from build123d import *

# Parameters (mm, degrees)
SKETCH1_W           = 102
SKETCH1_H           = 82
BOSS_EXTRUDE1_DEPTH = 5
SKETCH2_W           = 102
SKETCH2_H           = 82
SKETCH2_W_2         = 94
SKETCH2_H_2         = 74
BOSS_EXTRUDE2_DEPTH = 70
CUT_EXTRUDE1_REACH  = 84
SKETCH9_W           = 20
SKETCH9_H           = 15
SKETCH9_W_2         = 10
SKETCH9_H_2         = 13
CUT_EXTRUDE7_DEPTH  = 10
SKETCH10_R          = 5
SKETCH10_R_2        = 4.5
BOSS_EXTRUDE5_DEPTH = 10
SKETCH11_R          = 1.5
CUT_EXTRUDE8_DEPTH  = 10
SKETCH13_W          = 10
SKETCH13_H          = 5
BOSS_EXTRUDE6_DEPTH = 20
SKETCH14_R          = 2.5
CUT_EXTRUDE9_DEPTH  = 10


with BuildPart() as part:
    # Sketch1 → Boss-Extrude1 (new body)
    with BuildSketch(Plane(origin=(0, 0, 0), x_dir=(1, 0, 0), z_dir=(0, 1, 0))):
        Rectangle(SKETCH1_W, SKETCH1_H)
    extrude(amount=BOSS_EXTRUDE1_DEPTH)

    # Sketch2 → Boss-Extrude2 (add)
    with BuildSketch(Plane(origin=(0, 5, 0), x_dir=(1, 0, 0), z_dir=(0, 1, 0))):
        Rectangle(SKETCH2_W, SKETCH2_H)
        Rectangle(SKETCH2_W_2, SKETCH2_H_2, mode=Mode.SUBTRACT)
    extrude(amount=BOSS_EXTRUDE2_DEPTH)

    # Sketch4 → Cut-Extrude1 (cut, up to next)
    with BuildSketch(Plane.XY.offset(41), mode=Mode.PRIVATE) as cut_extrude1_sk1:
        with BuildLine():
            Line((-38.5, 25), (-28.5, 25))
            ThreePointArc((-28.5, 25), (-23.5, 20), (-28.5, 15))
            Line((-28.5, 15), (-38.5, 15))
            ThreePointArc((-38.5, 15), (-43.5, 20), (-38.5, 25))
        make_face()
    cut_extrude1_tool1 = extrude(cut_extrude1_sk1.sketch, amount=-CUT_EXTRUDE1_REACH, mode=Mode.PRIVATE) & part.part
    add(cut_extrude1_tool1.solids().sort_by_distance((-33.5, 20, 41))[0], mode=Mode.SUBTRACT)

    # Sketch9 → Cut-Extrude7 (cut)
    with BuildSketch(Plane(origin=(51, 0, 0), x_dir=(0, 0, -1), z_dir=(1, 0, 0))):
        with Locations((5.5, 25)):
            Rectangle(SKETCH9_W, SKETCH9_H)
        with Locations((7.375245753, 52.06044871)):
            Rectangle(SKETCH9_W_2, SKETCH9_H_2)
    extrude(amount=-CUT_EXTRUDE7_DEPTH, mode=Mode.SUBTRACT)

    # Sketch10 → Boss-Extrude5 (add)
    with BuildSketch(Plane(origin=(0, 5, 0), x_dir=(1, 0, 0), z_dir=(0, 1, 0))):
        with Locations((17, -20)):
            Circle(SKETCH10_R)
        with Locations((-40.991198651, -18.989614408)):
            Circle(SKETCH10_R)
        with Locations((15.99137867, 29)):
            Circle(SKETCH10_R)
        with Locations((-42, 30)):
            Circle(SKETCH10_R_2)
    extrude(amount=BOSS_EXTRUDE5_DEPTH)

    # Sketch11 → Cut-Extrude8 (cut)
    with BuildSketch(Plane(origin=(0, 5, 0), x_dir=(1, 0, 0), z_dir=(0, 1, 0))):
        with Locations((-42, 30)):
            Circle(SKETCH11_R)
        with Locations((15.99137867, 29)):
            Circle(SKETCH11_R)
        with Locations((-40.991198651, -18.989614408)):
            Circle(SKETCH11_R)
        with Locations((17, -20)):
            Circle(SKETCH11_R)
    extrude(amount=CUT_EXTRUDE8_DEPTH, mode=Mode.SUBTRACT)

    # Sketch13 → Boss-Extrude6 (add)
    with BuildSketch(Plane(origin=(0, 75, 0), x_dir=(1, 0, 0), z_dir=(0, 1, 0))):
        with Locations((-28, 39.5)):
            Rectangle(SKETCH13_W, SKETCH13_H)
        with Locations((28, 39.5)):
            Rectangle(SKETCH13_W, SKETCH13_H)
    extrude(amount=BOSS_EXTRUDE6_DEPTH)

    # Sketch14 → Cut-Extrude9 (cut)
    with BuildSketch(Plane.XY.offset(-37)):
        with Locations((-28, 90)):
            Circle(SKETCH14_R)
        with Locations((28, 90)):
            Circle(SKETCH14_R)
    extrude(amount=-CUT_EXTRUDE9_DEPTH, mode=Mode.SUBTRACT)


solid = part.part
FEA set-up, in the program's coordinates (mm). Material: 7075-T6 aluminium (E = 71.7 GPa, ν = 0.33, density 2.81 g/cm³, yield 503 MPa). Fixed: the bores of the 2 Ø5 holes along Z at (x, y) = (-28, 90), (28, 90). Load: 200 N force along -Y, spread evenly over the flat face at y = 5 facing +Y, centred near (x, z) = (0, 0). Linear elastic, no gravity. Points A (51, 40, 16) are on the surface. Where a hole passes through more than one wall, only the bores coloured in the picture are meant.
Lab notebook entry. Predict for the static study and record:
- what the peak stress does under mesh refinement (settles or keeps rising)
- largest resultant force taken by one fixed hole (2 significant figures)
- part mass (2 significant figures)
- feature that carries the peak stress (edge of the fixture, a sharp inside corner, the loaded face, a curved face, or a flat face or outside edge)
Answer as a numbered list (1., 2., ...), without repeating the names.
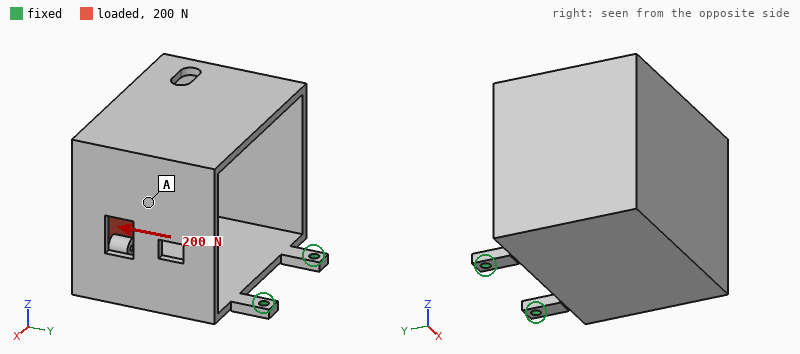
1. keeps rising
2. 100 N
3. 400 g
4. a sharp inside corner
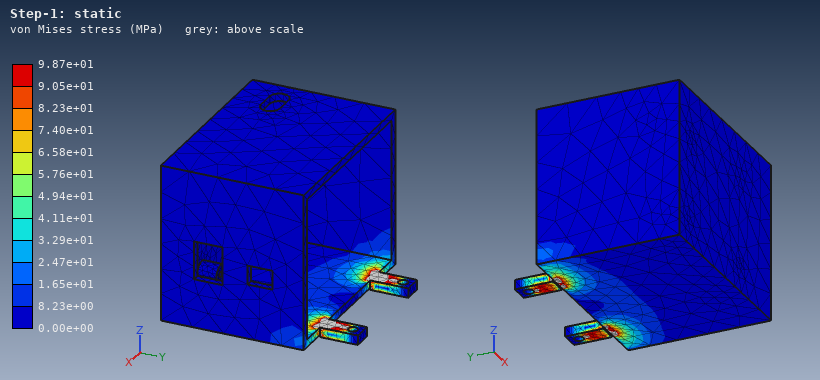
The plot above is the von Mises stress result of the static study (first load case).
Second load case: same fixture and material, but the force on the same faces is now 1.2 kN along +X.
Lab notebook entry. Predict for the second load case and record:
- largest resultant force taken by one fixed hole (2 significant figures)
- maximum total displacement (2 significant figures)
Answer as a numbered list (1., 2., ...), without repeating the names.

1. 1.8 kN
2. 1.8 mm
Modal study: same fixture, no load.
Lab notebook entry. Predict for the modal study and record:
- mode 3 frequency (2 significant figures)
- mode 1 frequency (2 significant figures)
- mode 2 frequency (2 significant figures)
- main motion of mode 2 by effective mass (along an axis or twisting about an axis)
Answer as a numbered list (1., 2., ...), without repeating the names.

1. 650 Hz
2. 80 Hz
3. 210 Hz
4. along X
